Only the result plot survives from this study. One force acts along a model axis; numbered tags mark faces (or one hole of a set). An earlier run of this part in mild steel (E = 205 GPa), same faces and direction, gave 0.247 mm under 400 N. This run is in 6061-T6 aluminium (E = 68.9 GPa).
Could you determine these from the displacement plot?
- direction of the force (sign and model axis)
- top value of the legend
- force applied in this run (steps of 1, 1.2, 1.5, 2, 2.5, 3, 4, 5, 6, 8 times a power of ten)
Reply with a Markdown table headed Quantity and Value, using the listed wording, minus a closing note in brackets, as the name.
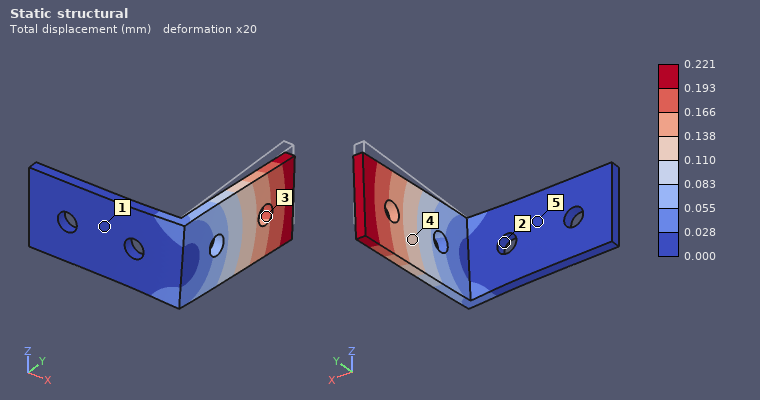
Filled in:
| Quantity | Value |
|---|---|
| direction of the force | -Z |
| top value of the legend | 0.221 mm |
| force applied in this run | 120 N |
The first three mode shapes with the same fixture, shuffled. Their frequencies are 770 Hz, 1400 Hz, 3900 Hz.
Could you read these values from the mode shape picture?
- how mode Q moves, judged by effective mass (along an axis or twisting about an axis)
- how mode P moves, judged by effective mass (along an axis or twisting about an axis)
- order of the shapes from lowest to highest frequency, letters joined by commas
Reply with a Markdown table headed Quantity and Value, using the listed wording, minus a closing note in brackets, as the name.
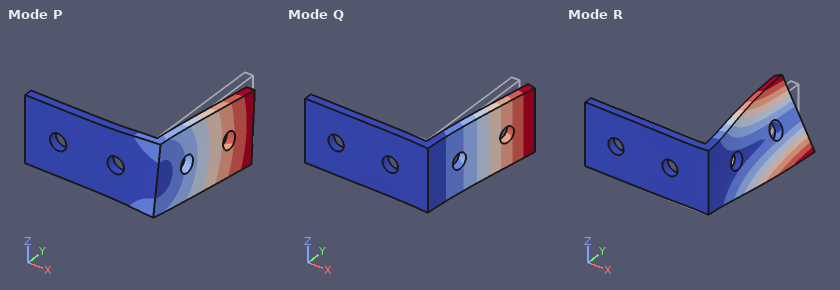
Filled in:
| Quantity | Value |
|---|---|
| how mode Q moves, judged by effective mass | along X |
| how mode P moves, judged by effective mass | along Z |
| order of the shapes from lowest to highest frequency, letters joined by commas | Q, P, R |
